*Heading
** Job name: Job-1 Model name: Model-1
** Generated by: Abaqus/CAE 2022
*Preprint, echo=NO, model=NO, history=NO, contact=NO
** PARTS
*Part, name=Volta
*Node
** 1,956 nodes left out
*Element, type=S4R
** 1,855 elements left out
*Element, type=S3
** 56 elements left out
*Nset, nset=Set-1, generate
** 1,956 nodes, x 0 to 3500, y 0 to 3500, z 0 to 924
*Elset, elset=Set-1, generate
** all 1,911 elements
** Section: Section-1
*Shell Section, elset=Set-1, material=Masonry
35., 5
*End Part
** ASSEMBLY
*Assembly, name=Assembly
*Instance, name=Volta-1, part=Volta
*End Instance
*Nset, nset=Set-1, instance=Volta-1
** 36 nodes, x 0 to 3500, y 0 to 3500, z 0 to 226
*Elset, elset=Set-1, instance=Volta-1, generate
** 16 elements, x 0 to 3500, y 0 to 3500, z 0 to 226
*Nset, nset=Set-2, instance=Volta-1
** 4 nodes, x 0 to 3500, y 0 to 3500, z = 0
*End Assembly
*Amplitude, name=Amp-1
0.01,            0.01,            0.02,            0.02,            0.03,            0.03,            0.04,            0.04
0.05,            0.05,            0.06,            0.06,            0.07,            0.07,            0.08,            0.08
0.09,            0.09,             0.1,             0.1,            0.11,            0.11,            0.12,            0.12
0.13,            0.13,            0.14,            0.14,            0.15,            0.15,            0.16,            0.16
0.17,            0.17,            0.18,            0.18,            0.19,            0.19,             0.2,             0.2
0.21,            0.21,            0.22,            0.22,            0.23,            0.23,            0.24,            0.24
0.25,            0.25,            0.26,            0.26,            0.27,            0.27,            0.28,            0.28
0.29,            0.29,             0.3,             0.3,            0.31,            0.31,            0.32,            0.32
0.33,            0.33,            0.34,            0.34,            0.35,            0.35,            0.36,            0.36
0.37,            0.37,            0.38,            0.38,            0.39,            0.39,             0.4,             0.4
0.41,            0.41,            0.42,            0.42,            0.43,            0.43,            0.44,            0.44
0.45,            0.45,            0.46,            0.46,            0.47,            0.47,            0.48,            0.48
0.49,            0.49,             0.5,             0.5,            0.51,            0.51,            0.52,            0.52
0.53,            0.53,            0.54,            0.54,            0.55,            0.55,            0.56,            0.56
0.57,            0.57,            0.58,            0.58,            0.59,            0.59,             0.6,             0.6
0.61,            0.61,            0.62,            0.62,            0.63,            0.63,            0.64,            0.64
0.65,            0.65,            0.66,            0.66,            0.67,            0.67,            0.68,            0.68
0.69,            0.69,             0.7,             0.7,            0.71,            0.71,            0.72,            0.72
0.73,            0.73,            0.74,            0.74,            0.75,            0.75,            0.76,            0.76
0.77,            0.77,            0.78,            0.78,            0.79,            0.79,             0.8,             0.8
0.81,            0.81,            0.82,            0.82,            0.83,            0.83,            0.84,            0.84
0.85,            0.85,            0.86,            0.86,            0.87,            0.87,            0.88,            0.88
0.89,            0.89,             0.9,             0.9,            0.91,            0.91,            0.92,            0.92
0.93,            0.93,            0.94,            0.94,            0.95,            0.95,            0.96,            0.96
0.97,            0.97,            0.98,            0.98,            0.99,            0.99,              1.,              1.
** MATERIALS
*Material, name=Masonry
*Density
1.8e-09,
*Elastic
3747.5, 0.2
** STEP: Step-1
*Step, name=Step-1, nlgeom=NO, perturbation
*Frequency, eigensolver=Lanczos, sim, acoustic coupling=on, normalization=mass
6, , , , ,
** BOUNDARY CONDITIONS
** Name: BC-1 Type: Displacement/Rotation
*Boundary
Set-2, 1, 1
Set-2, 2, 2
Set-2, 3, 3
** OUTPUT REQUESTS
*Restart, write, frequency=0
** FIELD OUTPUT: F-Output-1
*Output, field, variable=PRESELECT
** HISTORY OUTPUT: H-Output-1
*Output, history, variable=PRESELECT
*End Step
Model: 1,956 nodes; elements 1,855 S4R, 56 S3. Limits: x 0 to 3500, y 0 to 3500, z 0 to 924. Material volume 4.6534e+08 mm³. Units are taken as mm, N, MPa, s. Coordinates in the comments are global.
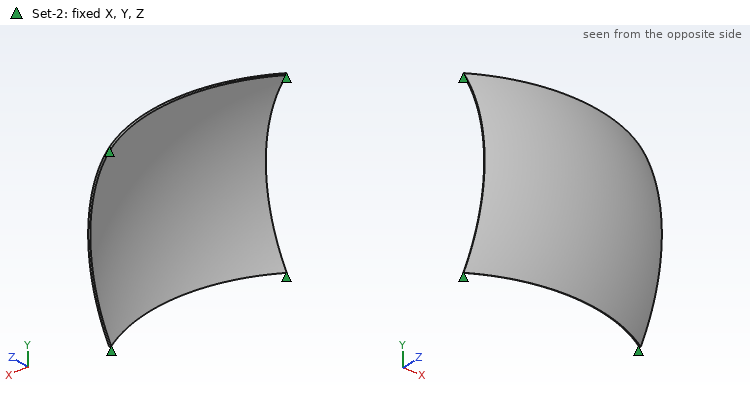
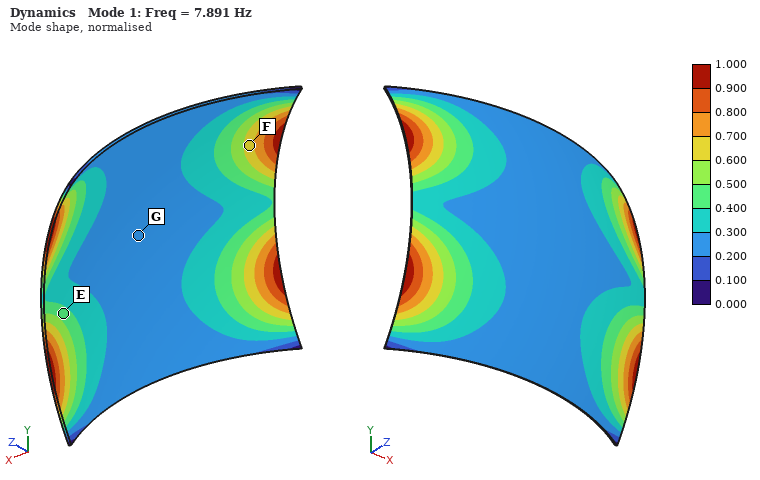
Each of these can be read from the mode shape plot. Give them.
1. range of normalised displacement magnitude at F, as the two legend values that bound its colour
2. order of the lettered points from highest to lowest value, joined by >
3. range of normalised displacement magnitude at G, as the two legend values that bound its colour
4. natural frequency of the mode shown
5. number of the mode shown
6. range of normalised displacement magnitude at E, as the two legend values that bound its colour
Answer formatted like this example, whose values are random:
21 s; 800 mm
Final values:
0.600 to 0.700; F > E > G; 0.200 to 0.300; 7.891 Hz; 1; 0.400 to 0.500
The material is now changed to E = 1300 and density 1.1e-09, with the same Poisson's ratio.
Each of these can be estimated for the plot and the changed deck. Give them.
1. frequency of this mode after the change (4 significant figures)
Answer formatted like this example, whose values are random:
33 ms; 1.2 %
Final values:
5.945 Hz
